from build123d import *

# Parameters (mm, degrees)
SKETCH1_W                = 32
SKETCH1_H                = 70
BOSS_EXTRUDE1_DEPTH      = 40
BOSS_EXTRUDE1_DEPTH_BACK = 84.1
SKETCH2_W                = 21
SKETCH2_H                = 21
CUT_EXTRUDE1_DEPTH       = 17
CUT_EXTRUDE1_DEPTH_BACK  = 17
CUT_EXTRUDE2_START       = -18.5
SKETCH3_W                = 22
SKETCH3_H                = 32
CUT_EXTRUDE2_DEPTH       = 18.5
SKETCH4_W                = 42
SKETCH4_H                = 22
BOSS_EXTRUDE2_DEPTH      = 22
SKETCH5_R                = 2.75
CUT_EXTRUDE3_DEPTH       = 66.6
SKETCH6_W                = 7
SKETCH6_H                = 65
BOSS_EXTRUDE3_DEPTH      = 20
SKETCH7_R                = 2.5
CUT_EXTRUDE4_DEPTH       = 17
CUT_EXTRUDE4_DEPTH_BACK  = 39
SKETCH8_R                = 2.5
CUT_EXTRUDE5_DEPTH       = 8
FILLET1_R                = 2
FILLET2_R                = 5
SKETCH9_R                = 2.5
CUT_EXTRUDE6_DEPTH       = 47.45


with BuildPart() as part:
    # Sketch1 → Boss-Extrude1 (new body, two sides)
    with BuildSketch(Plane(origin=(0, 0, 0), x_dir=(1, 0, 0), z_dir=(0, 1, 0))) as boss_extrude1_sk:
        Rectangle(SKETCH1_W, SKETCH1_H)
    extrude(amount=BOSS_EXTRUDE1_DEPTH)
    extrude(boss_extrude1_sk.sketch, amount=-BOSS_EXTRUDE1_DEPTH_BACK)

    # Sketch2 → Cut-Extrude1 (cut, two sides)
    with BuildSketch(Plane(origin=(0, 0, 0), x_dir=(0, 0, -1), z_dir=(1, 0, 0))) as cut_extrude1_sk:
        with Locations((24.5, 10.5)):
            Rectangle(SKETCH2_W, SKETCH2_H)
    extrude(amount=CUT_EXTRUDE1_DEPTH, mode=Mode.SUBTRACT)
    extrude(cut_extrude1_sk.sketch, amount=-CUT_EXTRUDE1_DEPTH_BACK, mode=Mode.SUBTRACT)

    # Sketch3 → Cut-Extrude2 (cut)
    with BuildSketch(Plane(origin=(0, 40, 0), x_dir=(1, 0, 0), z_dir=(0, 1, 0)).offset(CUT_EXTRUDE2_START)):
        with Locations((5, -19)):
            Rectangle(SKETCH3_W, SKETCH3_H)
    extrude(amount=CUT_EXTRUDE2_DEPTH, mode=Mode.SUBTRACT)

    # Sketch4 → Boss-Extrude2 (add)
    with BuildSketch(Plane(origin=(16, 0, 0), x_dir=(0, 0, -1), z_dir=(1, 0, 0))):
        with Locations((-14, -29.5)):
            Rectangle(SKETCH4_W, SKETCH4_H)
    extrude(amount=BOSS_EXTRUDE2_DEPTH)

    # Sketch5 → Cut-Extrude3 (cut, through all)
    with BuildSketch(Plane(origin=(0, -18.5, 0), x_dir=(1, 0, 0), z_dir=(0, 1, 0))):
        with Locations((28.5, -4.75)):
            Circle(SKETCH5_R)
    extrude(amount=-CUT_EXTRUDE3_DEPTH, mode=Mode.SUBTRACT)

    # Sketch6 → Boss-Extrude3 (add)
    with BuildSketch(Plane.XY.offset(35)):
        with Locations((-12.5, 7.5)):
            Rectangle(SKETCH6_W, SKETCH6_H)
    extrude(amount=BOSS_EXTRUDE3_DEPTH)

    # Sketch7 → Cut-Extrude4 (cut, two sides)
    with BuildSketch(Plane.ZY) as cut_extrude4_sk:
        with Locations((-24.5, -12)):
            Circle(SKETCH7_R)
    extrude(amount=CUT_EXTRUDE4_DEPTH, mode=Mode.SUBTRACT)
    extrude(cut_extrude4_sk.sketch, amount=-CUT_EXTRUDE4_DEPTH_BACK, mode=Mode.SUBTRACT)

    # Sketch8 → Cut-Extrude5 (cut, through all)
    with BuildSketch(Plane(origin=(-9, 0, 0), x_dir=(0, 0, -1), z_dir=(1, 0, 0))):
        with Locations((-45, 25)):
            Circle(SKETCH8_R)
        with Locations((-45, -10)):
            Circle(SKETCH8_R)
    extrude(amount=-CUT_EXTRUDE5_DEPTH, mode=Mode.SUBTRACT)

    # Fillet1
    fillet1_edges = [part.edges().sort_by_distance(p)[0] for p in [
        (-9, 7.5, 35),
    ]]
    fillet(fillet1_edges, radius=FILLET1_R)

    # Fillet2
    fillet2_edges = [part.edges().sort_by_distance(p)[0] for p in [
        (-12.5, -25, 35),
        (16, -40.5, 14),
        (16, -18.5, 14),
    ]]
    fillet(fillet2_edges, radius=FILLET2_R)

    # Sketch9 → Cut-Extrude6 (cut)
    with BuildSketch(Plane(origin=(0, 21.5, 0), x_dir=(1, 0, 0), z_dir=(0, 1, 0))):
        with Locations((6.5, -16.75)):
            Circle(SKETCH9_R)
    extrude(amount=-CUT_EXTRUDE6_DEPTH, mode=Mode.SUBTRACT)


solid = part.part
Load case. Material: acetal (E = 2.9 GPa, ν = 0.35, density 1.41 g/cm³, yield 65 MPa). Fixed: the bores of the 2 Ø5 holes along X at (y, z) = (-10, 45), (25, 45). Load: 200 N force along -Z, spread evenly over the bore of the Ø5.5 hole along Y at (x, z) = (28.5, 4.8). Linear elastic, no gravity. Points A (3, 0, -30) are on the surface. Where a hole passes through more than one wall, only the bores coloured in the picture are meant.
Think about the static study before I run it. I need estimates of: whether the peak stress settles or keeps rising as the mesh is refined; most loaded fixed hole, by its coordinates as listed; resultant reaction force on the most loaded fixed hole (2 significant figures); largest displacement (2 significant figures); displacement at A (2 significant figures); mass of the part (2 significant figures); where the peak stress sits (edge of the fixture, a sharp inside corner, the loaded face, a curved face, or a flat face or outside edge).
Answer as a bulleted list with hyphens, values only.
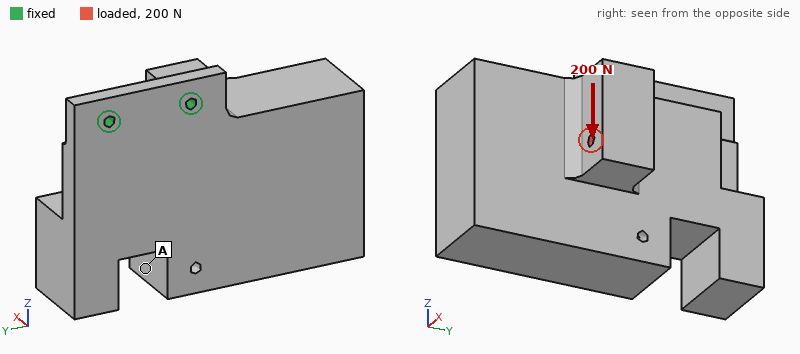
- keeps rising
- (-10, 45)
- 300 N
- 1.9 mm
- 1.6 mm
- 390 g
- edge of the fixture
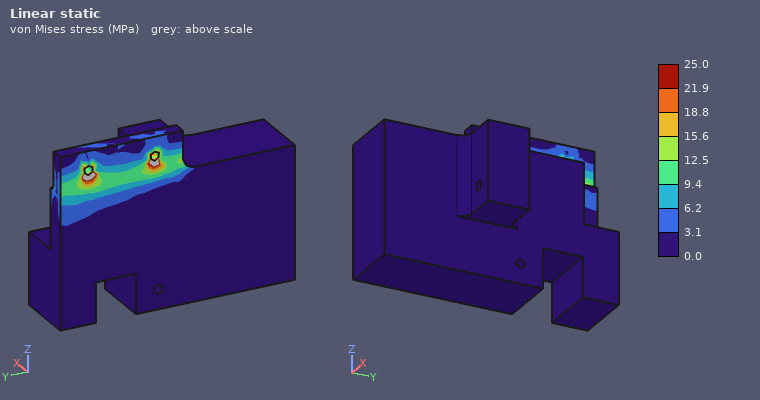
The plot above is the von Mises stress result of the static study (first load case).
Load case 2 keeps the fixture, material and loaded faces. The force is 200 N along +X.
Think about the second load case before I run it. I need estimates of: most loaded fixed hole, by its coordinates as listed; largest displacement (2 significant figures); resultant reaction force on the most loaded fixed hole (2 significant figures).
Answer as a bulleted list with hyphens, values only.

- (-10, 45)
- 1.8 mm
- 290 N
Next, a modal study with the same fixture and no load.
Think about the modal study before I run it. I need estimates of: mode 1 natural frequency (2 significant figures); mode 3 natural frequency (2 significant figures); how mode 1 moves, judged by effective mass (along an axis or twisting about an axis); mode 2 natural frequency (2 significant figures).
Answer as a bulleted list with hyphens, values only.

- 100 Hz
- 430 Hz
- along X
- 320 Hz
